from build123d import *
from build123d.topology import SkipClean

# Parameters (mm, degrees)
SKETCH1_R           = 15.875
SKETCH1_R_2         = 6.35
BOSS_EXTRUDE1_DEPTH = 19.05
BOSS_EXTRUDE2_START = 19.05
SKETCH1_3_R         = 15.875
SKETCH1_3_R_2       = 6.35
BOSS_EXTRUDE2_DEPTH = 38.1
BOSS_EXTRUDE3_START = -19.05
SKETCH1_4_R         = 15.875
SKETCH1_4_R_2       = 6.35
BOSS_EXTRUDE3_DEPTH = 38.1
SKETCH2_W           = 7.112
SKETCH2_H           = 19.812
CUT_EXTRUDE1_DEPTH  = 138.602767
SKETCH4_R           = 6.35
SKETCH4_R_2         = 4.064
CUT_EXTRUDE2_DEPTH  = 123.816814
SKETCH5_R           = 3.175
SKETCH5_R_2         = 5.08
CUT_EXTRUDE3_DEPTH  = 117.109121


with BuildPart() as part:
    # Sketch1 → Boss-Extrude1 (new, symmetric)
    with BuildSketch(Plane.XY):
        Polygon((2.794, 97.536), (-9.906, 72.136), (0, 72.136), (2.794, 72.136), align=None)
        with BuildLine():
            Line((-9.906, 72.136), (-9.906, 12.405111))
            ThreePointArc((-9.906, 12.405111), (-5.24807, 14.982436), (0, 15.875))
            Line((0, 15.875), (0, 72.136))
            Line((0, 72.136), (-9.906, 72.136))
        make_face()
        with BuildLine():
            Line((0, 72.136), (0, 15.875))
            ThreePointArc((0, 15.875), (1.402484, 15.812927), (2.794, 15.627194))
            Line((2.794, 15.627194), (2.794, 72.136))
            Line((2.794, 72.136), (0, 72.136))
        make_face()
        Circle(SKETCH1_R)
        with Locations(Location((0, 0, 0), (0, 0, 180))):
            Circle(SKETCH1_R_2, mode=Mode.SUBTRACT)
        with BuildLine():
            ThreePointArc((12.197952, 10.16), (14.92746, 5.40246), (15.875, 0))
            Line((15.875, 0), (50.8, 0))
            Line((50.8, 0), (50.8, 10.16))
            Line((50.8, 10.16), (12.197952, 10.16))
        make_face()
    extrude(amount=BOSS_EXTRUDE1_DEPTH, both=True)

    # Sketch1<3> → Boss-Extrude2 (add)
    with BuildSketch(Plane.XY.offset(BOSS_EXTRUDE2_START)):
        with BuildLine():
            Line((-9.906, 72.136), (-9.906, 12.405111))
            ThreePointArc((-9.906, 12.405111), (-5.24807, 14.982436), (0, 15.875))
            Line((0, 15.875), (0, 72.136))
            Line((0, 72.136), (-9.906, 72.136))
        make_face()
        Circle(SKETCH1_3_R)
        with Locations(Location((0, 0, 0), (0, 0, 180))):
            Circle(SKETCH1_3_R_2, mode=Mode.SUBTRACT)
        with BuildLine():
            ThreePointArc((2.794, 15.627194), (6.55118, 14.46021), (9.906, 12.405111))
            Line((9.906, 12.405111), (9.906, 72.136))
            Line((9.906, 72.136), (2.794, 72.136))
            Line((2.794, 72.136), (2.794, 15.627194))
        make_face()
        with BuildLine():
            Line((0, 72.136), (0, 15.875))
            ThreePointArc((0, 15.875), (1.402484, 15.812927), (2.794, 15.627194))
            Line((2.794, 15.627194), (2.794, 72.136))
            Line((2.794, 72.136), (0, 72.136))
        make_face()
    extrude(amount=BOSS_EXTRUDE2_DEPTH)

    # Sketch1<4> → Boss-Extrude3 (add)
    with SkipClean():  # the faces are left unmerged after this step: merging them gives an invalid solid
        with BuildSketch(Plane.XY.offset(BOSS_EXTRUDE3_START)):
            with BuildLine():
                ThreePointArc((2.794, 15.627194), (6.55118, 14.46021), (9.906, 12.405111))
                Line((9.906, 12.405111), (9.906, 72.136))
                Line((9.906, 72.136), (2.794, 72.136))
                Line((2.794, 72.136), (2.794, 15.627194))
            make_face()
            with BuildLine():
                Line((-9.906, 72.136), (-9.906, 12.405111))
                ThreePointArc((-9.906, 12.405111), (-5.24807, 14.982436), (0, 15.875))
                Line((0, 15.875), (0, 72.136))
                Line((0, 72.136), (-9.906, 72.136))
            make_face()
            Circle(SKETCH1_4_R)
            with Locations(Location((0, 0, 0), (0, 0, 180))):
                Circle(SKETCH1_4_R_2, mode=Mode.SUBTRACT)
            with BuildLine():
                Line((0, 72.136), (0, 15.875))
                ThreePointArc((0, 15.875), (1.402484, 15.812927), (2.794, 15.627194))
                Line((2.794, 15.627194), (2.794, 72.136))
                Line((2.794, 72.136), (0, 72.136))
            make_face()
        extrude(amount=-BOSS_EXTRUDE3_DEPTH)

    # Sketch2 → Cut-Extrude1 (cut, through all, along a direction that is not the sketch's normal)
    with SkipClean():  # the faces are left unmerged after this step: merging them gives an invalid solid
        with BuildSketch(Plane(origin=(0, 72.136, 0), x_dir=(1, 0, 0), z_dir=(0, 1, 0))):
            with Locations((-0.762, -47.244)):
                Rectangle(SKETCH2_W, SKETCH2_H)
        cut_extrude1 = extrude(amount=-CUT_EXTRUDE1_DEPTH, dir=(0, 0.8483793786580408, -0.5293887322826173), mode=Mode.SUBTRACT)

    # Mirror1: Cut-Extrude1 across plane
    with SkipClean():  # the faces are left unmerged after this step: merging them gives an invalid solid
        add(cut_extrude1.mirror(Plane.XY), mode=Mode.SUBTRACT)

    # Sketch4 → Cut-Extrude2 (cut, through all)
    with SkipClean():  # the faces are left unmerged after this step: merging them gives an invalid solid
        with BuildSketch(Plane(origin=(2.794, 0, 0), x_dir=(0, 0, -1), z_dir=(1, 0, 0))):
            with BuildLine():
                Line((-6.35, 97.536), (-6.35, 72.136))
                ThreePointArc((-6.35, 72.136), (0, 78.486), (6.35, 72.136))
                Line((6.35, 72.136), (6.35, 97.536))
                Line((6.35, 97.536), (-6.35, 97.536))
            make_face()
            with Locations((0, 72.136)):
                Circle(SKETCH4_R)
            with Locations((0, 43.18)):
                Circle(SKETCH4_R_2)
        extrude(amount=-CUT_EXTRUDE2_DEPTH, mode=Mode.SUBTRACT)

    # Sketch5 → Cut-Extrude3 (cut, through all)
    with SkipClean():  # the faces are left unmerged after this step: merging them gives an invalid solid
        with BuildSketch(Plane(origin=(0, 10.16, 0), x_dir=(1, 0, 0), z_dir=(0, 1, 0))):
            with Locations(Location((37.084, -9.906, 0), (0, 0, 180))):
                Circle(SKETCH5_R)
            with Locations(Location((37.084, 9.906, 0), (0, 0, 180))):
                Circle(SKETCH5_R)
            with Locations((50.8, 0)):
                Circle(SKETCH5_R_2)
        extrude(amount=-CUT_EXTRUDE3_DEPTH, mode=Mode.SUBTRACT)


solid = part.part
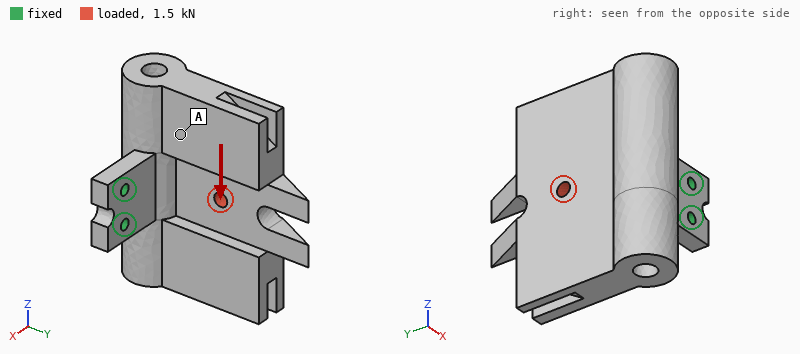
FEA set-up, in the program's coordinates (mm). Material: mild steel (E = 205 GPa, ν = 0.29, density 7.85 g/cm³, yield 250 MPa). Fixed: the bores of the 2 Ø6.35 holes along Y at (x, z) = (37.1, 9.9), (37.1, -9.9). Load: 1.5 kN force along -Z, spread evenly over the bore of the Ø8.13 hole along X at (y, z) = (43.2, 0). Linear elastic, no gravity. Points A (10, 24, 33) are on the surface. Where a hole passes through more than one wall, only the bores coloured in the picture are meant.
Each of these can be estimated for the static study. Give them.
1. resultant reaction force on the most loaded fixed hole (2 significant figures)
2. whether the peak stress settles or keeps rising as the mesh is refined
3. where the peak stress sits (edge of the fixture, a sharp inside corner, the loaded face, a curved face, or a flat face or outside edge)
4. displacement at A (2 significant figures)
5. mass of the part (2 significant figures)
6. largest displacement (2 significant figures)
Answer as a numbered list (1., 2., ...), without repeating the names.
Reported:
1. 3.3 kN
2. keeps rising
3. edge of the fixture
4. 35 µm
5. 1.6 kg
6. 86 µm
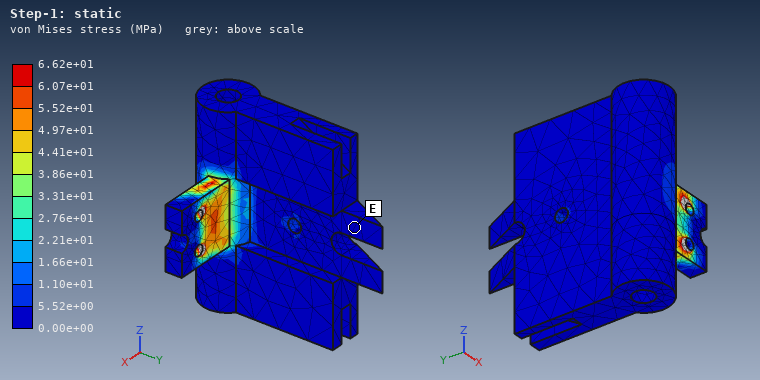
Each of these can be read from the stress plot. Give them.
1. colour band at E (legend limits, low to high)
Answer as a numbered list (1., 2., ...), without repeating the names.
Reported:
1. 0.00e+00 to 5.52e+00 MPa
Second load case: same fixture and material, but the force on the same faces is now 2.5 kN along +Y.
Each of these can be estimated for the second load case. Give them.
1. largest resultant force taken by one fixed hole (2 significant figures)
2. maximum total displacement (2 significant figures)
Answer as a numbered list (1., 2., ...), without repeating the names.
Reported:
1. 1.3 kN
2. 0.24 mm
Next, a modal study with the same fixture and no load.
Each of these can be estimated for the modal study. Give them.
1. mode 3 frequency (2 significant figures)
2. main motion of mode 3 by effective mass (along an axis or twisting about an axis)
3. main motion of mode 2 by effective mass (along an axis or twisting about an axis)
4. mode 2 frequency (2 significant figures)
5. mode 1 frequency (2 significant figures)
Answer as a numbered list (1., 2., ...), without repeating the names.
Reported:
1. 1600 Hz
2. along Z
3. along Z
4. 710 Hz
5. 510 Hz
